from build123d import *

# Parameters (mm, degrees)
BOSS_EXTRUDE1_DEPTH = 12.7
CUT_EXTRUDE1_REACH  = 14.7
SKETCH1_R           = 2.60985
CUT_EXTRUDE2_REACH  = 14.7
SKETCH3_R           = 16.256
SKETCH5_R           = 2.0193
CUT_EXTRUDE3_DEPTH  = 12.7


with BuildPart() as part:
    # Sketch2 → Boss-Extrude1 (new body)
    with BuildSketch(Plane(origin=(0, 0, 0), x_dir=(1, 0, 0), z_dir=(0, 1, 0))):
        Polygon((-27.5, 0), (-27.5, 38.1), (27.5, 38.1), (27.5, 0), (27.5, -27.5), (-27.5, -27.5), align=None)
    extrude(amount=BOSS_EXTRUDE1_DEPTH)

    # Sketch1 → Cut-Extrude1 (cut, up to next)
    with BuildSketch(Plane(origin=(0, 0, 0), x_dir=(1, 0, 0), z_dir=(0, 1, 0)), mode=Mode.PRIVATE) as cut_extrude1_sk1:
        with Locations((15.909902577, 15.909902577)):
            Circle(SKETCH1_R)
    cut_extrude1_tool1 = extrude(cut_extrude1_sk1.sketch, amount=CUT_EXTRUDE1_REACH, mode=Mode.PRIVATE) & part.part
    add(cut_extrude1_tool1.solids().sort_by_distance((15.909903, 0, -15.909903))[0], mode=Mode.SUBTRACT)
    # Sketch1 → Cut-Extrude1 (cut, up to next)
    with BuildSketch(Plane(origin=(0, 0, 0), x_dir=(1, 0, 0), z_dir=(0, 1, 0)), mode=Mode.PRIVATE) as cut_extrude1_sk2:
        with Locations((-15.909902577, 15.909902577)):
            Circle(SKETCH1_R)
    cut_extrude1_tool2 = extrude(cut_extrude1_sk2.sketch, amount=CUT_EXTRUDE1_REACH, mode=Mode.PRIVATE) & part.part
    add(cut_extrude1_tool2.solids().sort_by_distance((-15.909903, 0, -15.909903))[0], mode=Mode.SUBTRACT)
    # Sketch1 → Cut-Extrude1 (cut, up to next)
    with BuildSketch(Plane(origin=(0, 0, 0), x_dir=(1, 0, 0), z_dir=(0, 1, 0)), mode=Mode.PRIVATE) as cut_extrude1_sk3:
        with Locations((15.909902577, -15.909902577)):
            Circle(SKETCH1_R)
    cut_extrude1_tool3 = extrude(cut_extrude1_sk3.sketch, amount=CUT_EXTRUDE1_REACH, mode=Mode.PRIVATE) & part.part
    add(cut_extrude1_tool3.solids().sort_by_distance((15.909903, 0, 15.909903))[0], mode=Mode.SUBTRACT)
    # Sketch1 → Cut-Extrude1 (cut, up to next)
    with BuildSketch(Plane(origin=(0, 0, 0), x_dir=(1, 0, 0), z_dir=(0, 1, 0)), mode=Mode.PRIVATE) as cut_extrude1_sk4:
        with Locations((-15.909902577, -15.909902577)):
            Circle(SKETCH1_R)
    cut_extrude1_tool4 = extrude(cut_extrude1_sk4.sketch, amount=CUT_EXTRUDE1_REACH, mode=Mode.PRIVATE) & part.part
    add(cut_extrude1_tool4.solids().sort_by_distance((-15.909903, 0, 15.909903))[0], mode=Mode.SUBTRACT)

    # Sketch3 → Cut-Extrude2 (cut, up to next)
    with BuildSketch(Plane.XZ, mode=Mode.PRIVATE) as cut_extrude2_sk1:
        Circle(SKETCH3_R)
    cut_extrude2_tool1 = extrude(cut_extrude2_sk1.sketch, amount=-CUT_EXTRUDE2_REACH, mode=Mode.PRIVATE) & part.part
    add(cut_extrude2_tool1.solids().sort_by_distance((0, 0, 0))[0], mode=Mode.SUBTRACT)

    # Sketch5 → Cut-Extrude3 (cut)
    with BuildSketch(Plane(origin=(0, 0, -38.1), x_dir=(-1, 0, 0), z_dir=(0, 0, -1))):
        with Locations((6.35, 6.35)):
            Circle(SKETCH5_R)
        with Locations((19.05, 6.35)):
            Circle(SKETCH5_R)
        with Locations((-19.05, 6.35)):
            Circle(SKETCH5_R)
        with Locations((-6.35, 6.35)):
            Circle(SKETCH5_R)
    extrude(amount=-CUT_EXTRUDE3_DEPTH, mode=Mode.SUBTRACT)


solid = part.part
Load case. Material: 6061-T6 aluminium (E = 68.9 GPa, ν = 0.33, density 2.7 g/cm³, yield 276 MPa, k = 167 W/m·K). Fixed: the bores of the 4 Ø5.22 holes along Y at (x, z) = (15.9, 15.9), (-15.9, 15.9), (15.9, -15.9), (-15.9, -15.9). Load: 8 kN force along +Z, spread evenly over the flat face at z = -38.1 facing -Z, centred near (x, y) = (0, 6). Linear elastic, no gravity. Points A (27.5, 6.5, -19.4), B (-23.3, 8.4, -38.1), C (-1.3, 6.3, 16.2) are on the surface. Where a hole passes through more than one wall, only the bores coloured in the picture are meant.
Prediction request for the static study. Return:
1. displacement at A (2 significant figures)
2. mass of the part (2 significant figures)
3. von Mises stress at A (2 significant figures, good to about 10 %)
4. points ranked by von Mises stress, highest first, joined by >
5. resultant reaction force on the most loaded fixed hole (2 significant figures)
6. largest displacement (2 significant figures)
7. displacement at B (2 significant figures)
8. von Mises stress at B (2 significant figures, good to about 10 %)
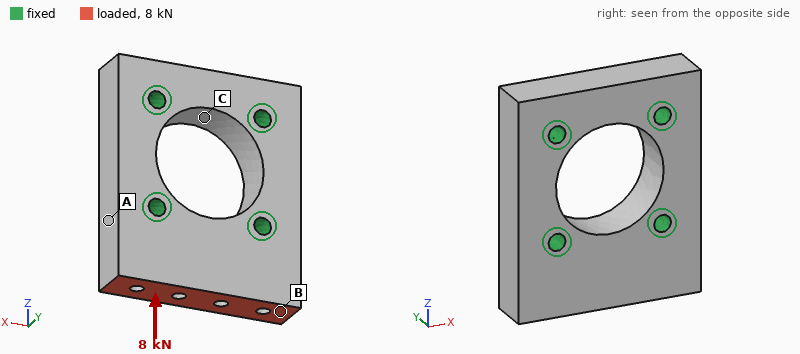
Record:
2.3 µm
91 g
7.4 MPa
B > A > C
3.8 kN
5.7 µm
5.0 µm
12 MPa
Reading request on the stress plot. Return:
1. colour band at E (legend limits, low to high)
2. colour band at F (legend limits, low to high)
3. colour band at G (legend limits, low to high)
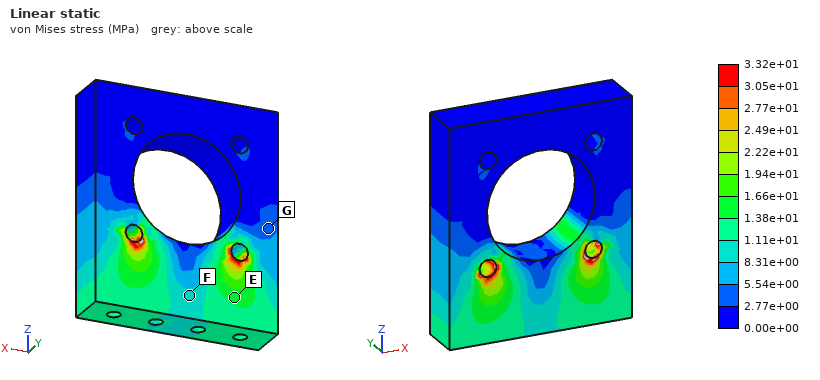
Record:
1.38e+01 to 1.66e+01 MPa
8.31e+00 to 1.11e+01 MPa
2.77e+00 to 5.54e+00 MPa
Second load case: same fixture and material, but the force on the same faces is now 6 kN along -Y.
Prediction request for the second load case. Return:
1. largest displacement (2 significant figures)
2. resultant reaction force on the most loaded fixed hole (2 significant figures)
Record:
66 µm
3.3 kN
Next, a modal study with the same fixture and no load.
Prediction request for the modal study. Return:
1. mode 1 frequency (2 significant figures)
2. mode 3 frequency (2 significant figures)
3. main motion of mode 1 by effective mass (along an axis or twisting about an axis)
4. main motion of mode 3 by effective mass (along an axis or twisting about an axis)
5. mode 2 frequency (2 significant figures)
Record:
15 kHz
26 kHz
along Y
along X
20 kHz
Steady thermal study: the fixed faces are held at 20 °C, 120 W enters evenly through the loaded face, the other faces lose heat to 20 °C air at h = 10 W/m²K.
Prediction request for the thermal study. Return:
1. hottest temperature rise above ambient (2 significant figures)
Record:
27 K
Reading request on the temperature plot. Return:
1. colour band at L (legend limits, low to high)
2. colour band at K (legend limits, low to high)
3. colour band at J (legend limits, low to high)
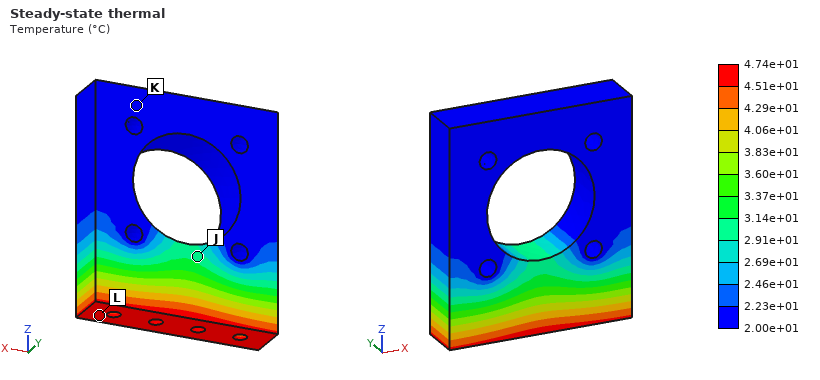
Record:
4.51e+01 to 4.74e+01 °C
2.00e+01 to 2.23e+01 °C
2.91e+01 to 3.14e+01 °C
